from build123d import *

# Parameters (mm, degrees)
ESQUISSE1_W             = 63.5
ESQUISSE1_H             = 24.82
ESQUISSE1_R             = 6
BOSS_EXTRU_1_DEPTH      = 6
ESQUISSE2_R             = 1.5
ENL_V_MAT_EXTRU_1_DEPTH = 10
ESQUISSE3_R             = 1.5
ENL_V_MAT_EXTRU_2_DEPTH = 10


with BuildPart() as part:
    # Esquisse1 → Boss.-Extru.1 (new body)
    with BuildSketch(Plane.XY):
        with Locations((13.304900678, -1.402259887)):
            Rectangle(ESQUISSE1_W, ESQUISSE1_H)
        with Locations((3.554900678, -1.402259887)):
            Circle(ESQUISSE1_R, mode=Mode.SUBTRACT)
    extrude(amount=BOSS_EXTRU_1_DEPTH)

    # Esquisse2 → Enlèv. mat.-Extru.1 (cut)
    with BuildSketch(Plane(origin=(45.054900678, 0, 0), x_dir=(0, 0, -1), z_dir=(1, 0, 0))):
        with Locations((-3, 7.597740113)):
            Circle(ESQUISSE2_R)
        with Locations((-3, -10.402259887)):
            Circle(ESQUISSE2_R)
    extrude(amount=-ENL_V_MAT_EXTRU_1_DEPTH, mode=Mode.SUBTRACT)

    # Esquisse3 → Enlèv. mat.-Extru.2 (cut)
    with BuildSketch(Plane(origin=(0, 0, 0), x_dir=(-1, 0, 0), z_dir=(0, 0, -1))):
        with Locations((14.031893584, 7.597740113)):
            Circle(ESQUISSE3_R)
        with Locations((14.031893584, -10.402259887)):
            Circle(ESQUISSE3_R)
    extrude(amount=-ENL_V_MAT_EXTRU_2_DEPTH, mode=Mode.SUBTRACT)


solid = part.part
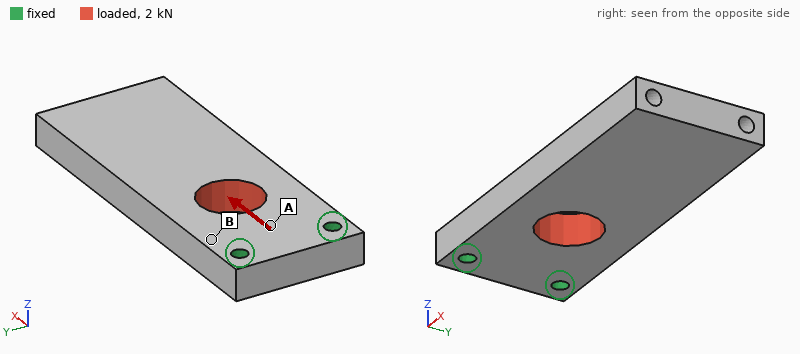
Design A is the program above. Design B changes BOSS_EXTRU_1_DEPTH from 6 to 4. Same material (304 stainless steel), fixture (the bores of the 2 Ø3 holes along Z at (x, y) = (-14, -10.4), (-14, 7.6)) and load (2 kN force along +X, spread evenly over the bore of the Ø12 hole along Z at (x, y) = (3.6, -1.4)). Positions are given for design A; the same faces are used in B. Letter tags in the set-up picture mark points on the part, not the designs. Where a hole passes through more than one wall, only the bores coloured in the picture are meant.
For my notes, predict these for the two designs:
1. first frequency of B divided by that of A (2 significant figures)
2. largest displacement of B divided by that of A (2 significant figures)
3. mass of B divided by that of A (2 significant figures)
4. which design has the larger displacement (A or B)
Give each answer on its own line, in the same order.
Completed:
0.69
1.5
0.66
B
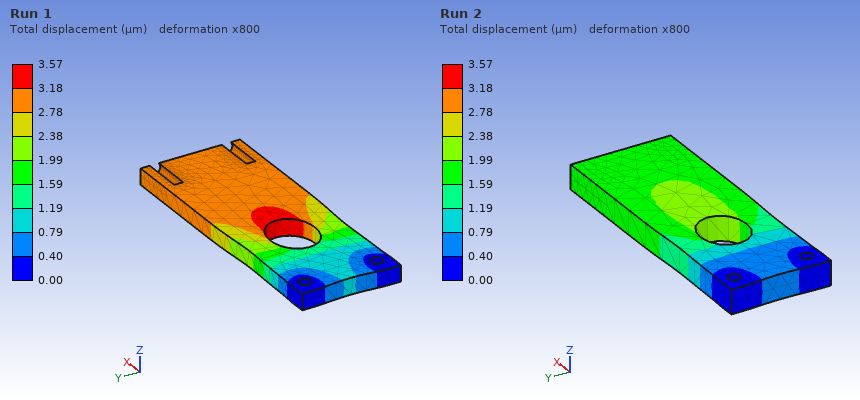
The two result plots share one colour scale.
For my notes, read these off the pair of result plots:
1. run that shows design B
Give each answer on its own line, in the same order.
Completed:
Run 1
